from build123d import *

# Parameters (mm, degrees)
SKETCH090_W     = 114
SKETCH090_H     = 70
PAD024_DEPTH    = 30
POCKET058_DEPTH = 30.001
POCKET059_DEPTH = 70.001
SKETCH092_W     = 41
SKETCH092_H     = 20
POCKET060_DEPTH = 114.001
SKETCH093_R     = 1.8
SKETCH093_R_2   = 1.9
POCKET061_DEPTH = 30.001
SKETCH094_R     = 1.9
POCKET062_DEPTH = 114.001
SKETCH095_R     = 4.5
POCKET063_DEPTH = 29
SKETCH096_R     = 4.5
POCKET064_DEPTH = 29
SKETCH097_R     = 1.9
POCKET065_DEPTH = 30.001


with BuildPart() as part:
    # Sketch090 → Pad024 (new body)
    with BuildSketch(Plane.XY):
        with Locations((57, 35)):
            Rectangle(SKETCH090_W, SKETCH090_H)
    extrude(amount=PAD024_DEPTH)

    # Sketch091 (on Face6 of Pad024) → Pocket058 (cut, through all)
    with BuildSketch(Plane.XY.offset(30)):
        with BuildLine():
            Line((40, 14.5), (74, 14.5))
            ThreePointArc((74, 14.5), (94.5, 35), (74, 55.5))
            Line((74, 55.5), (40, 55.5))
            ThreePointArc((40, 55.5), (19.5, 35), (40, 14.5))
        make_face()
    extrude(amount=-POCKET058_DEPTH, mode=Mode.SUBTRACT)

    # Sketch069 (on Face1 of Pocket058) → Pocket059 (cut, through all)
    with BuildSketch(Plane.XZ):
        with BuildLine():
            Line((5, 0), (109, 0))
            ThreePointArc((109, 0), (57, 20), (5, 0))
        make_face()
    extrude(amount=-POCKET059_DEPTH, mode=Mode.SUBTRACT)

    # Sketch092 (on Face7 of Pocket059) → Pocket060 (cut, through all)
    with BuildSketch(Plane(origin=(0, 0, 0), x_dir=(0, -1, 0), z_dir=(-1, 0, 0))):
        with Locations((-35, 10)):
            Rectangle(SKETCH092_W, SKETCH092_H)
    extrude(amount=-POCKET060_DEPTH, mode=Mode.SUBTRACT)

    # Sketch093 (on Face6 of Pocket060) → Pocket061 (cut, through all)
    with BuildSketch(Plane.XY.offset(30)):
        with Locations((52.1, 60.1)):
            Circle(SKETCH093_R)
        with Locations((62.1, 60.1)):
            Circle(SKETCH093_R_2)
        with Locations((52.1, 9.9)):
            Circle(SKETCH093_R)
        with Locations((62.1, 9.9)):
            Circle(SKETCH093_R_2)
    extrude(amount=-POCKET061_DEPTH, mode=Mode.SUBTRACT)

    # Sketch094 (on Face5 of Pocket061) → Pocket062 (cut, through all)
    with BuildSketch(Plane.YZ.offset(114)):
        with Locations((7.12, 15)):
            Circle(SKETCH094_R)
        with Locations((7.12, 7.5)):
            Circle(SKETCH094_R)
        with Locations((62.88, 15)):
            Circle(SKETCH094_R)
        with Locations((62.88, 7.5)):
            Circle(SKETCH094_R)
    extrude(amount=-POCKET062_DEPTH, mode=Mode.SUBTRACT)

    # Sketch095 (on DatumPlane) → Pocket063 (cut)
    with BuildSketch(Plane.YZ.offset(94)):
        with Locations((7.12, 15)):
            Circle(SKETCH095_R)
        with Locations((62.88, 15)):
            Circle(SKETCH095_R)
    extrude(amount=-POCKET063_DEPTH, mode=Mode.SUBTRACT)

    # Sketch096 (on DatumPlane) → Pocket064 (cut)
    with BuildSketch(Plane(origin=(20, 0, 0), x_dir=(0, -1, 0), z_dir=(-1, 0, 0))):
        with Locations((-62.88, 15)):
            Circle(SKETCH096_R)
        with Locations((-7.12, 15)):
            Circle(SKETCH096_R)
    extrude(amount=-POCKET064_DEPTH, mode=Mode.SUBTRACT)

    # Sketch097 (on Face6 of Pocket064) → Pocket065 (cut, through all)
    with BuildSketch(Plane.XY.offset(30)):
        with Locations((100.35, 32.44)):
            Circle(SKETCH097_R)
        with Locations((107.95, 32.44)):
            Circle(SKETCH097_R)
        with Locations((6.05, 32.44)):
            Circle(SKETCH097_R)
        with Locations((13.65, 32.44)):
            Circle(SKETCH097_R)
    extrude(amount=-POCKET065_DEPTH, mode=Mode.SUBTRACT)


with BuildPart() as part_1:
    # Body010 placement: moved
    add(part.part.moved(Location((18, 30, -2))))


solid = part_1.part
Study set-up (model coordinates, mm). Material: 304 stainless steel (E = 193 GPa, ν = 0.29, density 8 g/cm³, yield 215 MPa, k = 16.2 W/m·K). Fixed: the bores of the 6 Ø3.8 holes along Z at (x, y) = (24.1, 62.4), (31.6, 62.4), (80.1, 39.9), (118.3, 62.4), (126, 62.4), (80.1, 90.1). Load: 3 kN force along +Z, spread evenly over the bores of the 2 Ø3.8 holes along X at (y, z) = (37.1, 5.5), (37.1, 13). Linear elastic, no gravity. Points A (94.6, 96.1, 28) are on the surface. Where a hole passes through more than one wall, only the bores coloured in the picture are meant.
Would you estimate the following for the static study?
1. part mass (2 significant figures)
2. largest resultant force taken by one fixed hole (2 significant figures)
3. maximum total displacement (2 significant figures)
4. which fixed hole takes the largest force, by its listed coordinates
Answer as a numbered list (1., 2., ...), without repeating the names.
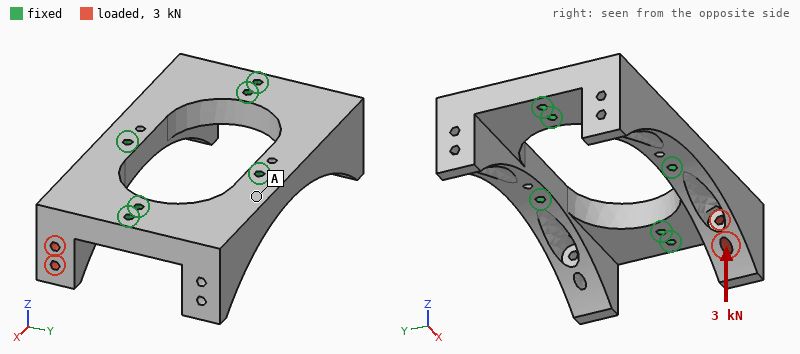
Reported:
1. 580 g
2. 1.9 kN
3. 63 µm
4. (126, 62.4)
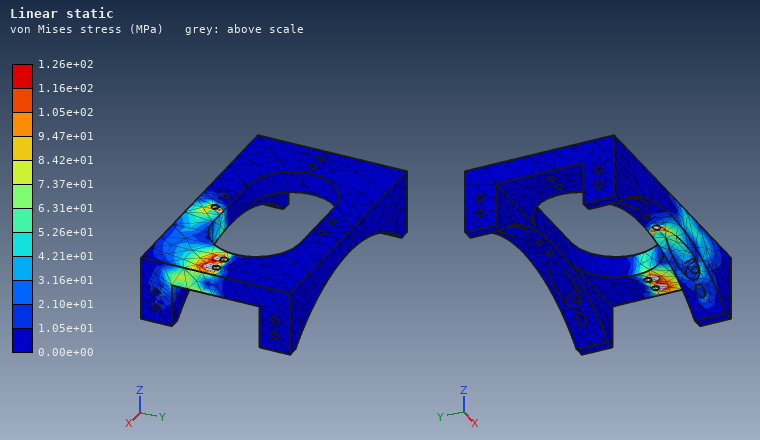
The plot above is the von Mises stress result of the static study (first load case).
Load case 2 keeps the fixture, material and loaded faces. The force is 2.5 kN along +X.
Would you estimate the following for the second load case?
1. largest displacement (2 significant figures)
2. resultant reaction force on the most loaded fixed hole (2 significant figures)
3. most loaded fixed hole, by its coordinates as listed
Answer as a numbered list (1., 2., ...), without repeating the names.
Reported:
1. 21 µm
2. 2.0 kN
3. (80.1, 39.9)
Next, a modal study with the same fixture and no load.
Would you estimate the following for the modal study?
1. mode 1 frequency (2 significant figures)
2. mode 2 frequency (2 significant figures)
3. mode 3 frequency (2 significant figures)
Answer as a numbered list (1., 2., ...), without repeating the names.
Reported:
1. 3900 Hz
2. 4400 Hz
3. 4700 Hz
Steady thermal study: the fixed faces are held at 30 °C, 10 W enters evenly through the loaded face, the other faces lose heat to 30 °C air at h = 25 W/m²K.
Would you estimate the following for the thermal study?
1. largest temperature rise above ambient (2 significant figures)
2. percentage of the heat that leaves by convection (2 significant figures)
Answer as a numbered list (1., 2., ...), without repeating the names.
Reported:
1. 54 K
2. 31 %
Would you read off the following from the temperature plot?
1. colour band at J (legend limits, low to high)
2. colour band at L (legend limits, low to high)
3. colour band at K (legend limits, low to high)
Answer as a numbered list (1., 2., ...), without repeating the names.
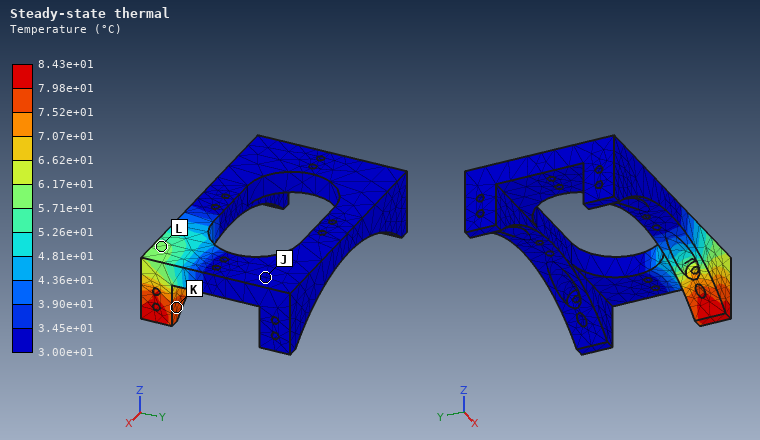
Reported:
1. 3.00e+01 to 3.45e+01 °C
2. 5.71e+01 to 6.17e+01 °C
3. 7.52e+01 to 7.98e+01 °C
